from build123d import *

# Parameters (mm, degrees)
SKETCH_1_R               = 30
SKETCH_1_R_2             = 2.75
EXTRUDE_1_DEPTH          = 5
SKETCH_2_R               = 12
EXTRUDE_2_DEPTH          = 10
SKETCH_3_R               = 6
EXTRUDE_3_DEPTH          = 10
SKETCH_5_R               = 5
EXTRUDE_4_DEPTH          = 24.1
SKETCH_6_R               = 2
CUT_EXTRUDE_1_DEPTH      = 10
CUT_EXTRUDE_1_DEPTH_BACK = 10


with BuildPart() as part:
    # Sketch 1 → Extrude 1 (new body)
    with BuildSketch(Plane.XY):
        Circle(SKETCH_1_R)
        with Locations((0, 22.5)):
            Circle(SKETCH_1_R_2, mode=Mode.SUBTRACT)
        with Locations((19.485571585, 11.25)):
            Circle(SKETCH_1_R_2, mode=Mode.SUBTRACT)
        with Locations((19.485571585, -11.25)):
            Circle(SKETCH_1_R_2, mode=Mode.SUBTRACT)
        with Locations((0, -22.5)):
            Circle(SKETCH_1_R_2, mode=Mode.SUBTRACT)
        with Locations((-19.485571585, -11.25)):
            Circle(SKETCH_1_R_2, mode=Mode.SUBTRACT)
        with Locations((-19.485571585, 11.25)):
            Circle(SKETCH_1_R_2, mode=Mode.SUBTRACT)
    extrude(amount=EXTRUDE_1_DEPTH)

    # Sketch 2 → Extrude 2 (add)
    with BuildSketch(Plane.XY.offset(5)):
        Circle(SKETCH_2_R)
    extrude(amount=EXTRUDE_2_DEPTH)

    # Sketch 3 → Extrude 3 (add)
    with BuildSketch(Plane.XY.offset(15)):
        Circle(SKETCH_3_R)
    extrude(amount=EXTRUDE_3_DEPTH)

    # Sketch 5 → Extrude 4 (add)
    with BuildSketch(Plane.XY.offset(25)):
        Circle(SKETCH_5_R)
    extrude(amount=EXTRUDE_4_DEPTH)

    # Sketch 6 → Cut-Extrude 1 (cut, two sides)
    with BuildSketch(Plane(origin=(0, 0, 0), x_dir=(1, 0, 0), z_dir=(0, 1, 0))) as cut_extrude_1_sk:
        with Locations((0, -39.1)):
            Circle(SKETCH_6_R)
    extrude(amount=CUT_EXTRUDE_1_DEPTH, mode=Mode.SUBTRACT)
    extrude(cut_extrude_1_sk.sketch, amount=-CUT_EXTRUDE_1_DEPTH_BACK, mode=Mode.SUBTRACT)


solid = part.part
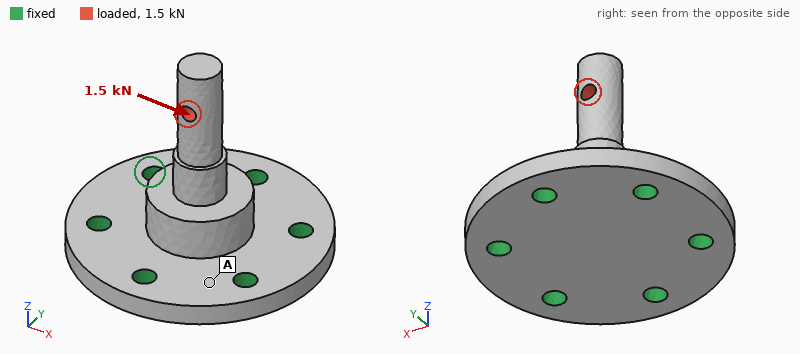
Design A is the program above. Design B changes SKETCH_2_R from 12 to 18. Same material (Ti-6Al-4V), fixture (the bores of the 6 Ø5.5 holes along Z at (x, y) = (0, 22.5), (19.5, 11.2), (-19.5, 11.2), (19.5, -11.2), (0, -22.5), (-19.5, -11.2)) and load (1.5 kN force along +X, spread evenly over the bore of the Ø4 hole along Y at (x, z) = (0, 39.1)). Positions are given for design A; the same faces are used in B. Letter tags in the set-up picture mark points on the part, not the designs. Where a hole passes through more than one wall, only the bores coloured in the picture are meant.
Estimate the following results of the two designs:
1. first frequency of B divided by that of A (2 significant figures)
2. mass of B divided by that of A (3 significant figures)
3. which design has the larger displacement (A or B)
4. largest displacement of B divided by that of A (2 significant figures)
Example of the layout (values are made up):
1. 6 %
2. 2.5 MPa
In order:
1. 1.1
2. 1.27
3. A
4. 0.88
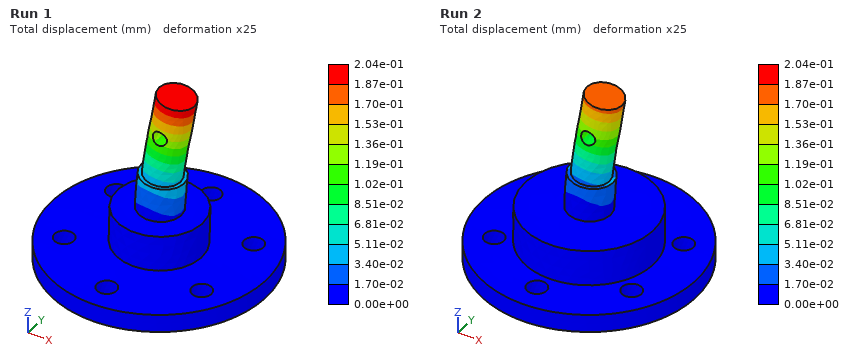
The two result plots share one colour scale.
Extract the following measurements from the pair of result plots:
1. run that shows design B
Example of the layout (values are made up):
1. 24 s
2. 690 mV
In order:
1. Run 2
